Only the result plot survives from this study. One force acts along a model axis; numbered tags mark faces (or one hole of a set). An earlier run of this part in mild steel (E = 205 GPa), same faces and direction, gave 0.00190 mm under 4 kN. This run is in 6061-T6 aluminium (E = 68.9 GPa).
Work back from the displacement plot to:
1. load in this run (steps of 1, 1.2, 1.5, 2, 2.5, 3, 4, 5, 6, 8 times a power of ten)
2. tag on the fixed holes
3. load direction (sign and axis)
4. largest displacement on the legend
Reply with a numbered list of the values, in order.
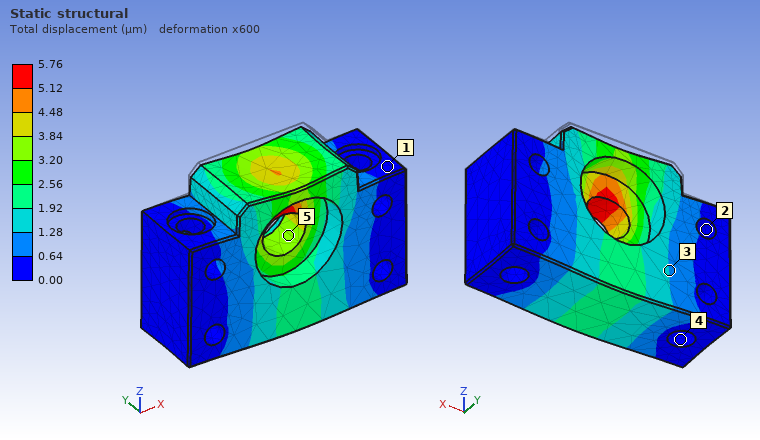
1. 4 kN
2. 4
3. -Z
4. 5.76 µm
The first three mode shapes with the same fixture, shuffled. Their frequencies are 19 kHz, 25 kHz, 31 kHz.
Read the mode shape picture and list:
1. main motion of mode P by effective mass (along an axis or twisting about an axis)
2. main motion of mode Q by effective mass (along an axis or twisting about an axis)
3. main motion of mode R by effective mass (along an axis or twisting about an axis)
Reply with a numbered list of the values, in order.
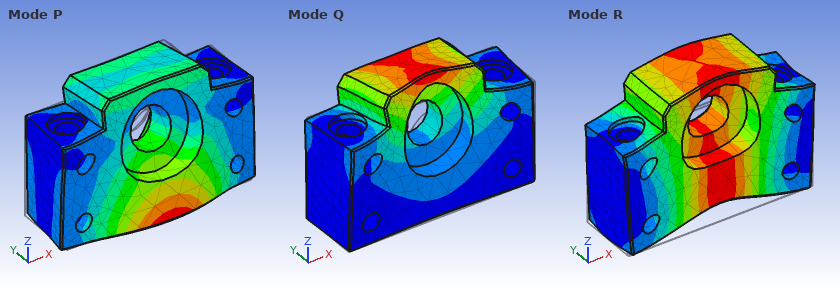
1. along Y
2. along Y
3. along Z
